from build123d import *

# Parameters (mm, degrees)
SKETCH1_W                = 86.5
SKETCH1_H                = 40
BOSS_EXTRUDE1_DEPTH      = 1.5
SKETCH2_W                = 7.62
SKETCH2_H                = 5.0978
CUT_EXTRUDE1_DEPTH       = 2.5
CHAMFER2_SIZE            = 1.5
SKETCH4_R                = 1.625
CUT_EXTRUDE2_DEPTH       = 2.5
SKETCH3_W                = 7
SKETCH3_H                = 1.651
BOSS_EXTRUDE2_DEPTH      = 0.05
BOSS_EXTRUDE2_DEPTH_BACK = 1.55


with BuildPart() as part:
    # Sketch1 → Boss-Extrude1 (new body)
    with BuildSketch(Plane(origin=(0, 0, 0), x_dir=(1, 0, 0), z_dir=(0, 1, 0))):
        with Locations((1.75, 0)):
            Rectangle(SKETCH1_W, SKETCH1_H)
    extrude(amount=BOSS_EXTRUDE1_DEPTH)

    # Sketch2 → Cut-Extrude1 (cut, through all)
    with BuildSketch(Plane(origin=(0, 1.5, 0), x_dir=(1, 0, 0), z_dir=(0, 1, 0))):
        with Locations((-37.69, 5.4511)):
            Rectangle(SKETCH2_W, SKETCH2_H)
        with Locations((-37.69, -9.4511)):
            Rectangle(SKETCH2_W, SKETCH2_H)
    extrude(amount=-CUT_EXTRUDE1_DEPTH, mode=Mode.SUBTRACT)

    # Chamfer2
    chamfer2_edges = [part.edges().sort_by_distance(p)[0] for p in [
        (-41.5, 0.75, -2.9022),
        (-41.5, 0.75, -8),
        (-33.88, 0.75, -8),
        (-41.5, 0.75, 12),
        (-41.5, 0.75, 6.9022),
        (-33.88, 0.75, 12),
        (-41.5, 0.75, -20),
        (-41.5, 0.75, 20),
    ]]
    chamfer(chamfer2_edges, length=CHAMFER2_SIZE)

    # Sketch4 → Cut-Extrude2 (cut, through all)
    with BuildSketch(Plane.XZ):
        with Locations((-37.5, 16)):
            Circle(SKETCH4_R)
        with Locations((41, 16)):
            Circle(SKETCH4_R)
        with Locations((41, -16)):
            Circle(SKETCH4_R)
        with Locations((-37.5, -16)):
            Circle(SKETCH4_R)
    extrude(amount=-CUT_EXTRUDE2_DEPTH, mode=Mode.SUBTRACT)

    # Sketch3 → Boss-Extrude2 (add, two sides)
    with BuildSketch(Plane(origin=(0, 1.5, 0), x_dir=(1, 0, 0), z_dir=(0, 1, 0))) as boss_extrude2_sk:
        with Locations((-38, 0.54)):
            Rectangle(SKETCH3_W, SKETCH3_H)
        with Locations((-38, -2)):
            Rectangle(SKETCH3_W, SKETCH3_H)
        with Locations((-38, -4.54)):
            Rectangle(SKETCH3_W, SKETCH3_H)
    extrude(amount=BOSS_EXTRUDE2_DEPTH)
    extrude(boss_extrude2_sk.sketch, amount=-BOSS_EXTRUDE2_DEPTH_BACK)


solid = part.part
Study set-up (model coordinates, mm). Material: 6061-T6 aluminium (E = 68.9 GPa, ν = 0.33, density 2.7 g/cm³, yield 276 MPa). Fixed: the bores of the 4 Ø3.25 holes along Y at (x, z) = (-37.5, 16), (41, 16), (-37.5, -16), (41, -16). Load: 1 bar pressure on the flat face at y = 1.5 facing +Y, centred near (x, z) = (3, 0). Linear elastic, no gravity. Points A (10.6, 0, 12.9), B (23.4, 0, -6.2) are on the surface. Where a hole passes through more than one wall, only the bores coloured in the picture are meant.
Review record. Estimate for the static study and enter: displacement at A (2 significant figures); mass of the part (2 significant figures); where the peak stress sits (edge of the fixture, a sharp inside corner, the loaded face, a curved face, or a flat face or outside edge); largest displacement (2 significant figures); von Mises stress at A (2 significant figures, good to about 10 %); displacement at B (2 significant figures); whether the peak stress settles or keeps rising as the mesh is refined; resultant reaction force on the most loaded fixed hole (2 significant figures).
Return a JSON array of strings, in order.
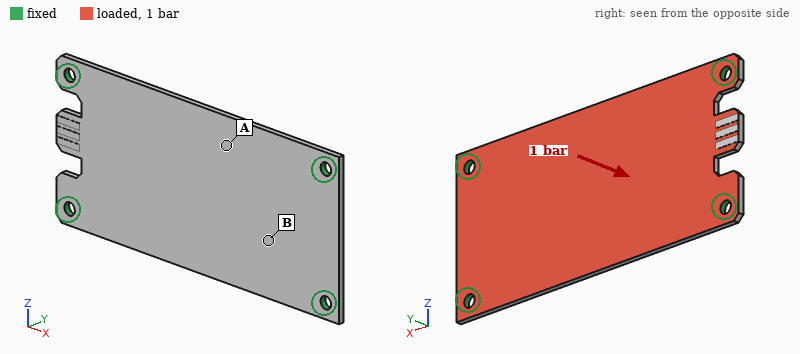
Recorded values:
["0.53 mm", "14 g", "edge of the fixture", "0.61 mm", "62 MPa", "0.30 mm", "keeps rising", "87 N"]
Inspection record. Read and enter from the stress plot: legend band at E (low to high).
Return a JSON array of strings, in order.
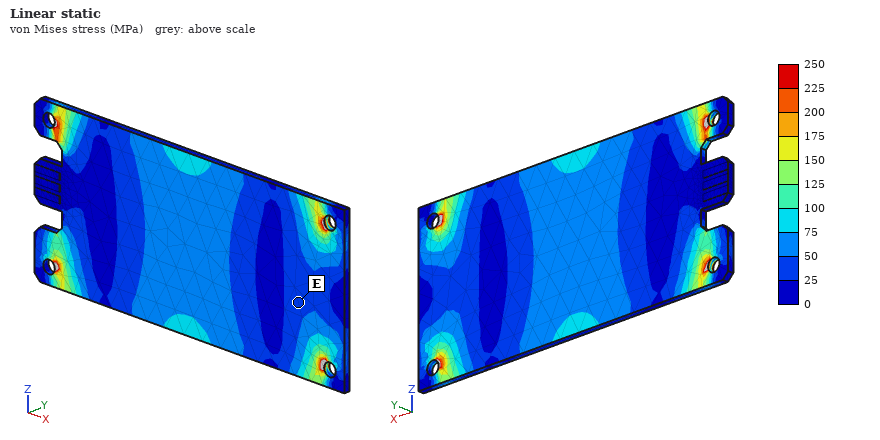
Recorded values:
["25 to 50 MPa"]
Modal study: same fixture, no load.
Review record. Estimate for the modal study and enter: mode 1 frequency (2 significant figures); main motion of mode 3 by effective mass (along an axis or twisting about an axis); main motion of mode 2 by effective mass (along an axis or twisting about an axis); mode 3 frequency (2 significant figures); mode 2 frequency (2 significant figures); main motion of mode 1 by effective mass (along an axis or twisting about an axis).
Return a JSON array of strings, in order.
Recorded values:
["1200 Hz", "twisting about Z", "twisting about X", "3300 Hz", "2100 Hz", "along Y"]
